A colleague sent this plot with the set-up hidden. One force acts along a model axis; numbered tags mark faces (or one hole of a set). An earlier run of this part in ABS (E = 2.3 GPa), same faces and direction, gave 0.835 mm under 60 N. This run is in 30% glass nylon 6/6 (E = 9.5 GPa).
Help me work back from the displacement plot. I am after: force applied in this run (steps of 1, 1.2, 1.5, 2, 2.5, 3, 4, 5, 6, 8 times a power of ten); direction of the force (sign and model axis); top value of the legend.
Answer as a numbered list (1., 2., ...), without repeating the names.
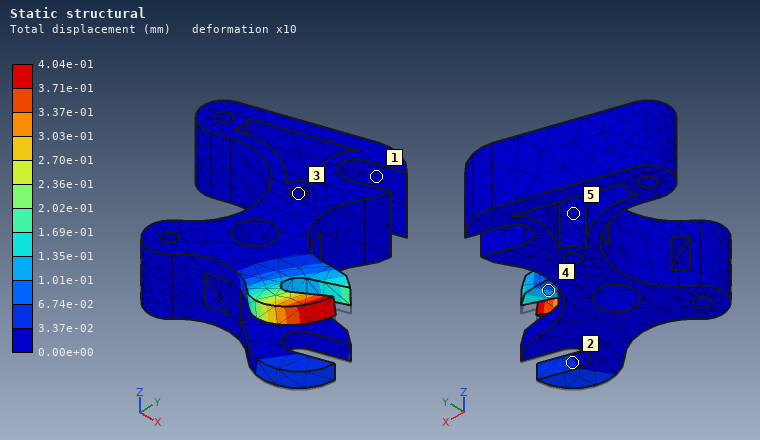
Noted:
1. 120 N
2. +Z
3. 4.04e-01 mm
